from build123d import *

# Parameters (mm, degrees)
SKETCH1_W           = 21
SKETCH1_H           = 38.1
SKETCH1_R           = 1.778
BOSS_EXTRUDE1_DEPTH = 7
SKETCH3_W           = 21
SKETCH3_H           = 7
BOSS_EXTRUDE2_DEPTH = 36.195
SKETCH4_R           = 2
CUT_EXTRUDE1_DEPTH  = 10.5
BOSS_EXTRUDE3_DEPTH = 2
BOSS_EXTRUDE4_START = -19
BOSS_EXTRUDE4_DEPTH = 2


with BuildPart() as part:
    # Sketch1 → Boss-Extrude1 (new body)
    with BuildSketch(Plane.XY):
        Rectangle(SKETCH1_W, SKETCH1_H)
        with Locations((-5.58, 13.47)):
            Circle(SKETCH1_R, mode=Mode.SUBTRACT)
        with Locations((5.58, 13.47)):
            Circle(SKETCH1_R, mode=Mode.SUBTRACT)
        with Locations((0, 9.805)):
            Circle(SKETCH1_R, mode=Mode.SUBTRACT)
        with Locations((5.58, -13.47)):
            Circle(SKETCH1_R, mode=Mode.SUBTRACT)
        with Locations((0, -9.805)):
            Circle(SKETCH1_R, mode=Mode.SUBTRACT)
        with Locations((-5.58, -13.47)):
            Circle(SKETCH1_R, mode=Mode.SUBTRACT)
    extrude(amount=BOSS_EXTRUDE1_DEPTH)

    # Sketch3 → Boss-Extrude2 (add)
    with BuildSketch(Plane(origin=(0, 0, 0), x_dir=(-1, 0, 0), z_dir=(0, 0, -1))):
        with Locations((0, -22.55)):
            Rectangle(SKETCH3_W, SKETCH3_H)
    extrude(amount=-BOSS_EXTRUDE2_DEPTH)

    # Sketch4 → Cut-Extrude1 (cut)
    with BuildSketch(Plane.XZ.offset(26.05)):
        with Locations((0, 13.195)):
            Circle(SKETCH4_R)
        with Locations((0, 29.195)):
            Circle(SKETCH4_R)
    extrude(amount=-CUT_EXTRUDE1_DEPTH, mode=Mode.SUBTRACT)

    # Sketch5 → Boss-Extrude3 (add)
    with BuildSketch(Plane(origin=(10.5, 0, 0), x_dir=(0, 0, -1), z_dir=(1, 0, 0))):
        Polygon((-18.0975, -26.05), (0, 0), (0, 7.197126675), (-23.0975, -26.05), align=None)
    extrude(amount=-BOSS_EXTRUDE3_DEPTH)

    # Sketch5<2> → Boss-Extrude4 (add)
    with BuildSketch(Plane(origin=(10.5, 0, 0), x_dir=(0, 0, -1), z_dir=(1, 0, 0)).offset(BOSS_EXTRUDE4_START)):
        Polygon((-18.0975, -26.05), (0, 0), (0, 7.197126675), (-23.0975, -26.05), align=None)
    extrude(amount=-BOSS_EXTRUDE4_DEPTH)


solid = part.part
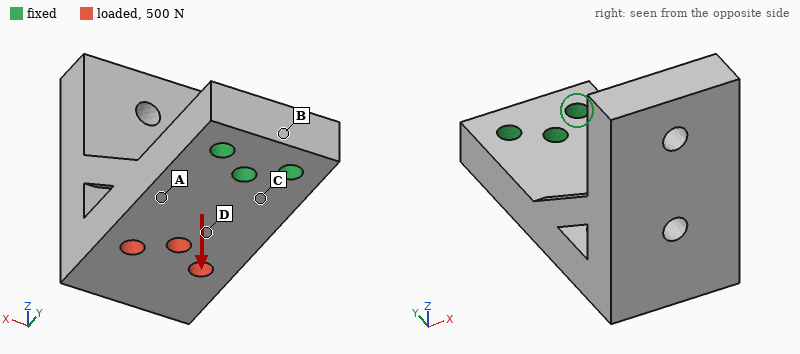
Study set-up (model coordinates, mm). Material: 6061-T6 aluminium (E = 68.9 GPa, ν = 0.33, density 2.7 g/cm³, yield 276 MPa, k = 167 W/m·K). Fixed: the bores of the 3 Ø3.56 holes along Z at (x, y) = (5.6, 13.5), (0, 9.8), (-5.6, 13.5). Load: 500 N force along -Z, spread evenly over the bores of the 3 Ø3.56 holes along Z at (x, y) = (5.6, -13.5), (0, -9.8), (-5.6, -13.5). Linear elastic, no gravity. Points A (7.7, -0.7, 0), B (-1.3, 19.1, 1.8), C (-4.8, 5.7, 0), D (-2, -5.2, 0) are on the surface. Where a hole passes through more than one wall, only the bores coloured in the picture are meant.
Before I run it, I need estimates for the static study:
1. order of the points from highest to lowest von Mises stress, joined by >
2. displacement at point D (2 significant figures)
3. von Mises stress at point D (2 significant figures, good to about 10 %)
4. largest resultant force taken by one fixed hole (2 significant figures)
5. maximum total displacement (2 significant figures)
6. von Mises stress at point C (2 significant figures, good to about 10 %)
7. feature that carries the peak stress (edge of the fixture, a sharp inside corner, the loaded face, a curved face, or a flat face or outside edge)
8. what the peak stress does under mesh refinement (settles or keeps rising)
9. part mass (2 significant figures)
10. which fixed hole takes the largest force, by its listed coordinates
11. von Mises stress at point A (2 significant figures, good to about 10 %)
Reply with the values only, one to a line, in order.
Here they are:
C > A > D > B
0.029 mm
19 MPa
740 N
0.13 mm
45 MPa
edge of the fixture
keeps rising
29 g
(0, 9.8)
33 MPa
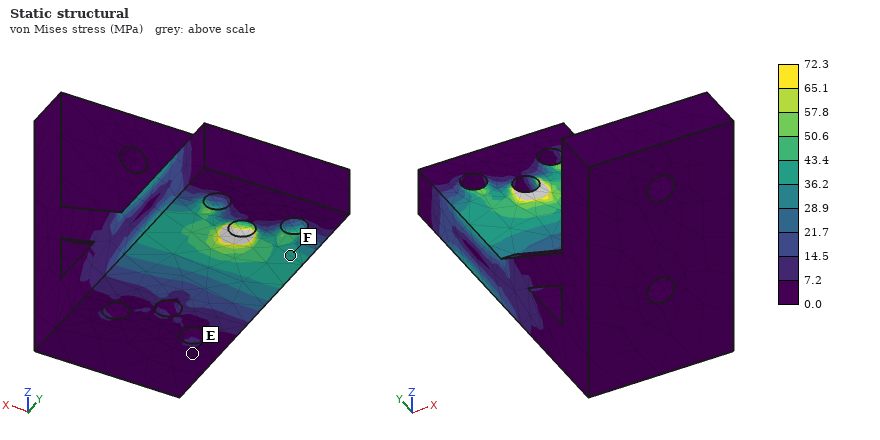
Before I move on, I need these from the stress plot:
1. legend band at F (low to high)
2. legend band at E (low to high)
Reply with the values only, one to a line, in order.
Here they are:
36.2 to 43.4 MPa
0.0 to 7.2 MPa
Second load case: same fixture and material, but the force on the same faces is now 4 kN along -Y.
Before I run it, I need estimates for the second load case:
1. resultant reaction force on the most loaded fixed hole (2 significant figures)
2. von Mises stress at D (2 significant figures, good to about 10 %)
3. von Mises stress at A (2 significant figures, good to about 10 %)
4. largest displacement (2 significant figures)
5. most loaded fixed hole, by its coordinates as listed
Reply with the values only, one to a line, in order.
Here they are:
1.7 kN
34 MPa
25 MPa
12 µm
(0, 9.8)
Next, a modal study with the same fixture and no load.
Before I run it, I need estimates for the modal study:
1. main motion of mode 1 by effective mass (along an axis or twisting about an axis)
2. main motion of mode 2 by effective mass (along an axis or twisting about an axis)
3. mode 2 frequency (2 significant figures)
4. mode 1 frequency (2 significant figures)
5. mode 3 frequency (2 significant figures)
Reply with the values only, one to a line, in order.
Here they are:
along Z
along X
2800 Hz
1900 Hz
6700 Hz
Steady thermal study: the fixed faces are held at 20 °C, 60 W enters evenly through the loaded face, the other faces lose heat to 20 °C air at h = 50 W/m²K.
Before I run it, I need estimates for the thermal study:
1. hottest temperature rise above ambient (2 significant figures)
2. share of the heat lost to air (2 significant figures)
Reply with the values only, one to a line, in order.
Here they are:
52 K
14 %
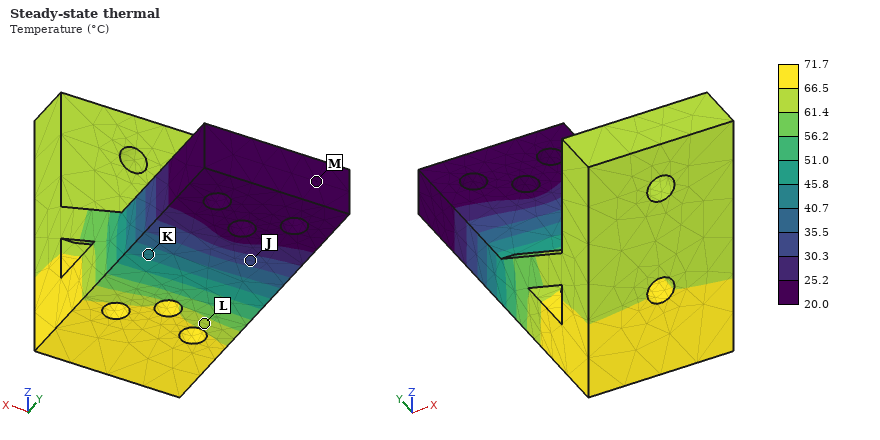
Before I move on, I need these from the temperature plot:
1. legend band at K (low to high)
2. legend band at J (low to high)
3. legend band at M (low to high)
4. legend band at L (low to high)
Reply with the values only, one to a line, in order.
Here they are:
40.7 to 45.8 °C
30.3 to 35.5 °C
20.0 to 25.2 °C
61.4 to 66.5 °C
